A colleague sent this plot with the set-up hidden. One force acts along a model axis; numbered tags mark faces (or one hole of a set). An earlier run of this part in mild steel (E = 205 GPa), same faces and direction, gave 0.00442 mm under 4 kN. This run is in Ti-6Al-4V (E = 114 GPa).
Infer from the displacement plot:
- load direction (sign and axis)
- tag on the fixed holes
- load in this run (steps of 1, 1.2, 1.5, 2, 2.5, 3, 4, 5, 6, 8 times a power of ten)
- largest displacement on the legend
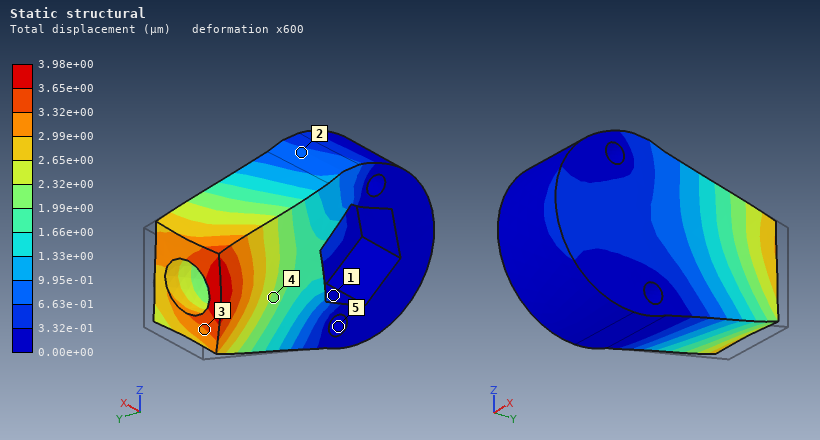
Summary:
-Y
5
2 kN
3.98e+00 µm
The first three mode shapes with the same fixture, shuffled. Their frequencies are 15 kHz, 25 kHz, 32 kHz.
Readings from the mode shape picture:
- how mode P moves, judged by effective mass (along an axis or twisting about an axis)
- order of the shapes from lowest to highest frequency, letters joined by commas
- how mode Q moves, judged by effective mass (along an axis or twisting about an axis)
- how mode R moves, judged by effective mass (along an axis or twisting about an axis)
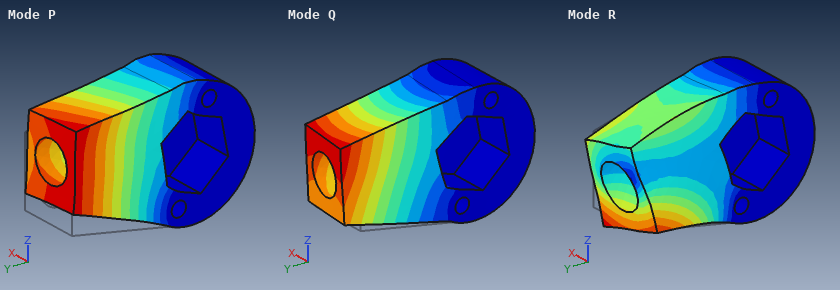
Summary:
along Z
Q, P, R
along X
twisting about Y
